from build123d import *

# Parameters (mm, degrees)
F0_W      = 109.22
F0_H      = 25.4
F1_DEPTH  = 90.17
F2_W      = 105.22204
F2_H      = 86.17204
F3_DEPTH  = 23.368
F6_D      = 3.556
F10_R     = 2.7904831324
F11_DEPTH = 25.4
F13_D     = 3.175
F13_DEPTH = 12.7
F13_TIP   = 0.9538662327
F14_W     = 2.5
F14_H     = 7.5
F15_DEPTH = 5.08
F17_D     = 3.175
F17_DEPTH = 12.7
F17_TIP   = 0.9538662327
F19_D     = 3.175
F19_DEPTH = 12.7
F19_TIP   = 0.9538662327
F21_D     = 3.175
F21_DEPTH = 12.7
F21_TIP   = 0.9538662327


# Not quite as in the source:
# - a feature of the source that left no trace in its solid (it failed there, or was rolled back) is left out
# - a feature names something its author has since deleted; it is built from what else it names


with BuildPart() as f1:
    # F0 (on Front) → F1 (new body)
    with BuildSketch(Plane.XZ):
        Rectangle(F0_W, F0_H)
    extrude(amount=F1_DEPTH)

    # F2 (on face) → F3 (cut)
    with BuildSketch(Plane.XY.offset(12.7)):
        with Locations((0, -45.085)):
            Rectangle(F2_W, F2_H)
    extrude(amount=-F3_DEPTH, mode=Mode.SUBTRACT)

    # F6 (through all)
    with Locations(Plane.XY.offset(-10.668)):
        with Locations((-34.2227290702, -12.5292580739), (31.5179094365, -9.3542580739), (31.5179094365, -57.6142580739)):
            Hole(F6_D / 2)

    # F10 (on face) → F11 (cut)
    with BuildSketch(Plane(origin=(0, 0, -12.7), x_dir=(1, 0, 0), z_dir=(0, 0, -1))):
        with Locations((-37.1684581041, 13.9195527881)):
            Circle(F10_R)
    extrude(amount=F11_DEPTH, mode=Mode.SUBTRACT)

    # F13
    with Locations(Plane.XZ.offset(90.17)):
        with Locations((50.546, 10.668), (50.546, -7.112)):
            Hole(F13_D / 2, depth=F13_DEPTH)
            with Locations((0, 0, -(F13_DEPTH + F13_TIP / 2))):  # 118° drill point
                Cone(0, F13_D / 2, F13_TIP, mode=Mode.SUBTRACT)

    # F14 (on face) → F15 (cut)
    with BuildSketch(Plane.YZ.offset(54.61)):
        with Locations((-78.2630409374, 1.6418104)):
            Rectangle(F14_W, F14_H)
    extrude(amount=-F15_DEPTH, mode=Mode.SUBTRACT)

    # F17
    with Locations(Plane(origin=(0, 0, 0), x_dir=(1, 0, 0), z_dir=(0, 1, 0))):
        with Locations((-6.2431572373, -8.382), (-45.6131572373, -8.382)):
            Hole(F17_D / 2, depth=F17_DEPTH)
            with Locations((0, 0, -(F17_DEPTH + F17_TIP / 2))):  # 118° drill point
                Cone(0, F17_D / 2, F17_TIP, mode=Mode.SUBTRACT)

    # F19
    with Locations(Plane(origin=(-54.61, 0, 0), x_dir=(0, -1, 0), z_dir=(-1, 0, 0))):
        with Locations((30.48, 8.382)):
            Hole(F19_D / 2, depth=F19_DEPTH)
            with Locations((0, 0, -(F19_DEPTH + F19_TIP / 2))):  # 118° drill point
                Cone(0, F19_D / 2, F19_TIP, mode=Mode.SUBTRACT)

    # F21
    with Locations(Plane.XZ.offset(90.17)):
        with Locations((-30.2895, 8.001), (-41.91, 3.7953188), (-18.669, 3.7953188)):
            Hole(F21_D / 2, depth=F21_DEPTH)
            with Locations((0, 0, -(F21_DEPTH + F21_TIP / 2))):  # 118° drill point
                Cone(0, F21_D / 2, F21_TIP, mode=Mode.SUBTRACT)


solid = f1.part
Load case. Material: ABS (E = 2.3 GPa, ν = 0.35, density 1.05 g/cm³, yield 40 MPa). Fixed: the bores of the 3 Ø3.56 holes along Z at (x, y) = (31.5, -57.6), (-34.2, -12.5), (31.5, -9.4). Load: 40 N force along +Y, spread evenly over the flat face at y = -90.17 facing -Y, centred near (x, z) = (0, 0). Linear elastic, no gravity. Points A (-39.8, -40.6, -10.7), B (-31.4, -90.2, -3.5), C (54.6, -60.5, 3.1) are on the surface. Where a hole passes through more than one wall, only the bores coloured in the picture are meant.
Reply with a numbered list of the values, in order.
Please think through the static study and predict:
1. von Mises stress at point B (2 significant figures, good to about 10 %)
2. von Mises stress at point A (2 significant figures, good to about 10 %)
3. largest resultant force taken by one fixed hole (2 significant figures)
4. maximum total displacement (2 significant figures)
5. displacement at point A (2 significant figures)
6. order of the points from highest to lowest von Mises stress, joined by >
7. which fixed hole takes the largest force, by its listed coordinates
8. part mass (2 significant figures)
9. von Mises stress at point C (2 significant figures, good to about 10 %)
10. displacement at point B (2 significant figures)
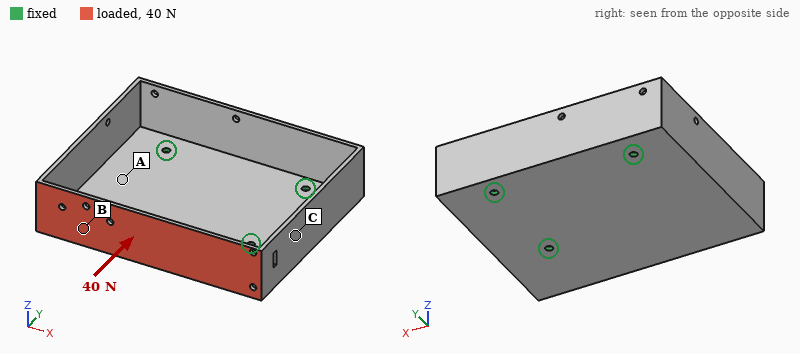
1. 2.3 MPa
2. 0.66 MPa
3. 20 N
4. 1.4 mm
5. 0.35 mm
6. B > C > A
7. (-34.2, -12.5)
8. 40 g
9. 1.4 MPa
10. 1.1 mm
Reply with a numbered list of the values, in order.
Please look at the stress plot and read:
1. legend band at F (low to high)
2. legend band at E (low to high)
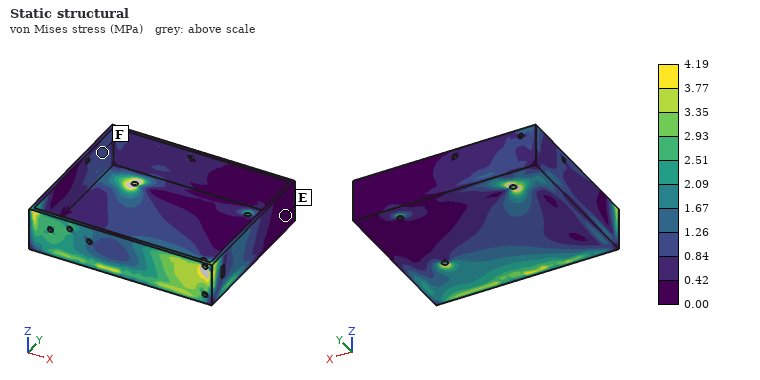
1. 0.84 to 1.26 MPa
2. 0.00 to 0.42 MPa
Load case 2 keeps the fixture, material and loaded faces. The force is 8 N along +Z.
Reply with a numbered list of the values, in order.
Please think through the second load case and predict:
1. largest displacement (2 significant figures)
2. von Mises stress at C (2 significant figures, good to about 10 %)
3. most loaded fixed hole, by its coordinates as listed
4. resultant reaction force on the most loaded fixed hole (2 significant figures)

1. 1.6 mm
2. 1.0 MPa
3. (31.5, -57.6)
4. 9.1 N
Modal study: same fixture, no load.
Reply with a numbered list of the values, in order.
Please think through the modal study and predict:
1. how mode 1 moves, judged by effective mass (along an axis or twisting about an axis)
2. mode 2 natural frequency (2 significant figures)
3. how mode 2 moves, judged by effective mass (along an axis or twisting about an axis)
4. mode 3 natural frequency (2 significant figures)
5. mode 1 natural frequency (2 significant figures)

1. along Z
2. 300 Hz
3. along Z
4. 540 Hz
5. 110 Hz
